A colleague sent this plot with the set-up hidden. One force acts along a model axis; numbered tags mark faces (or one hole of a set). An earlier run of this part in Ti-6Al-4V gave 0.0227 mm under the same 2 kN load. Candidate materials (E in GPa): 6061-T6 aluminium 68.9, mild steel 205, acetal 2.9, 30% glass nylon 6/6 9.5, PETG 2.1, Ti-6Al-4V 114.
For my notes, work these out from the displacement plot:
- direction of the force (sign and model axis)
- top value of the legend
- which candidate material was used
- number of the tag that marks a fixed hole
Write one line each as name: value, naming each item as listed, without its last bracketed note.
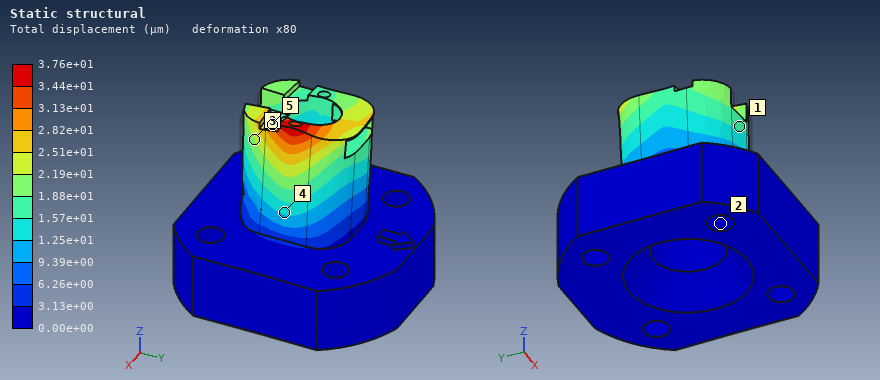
direction of the force: -X
top value of the legend: 3.76e+01 µm
which candidate material was used: 6061-T6 aluminium
number of the tag that marks a fixed hole: 2
